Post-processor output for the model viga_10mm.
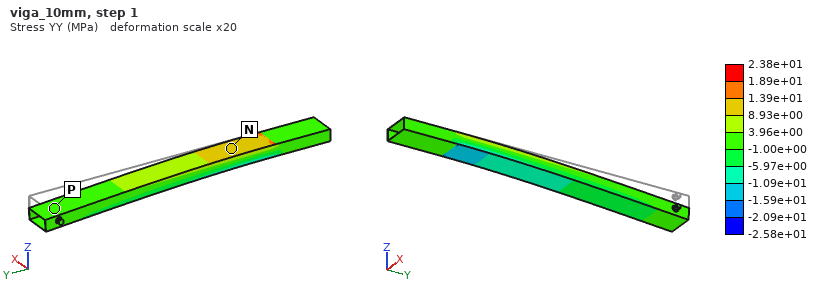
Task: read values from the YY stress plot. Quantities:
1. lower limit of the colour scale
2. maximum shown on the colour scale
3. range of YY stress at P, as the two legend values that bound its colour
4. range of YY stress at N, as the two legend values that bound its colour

-2.58e+01 MPa
2.38e+01 MPa
-1.00e+00 to 3.96e+00 MPa
8.93e+00 to 1.39e+01 MPa
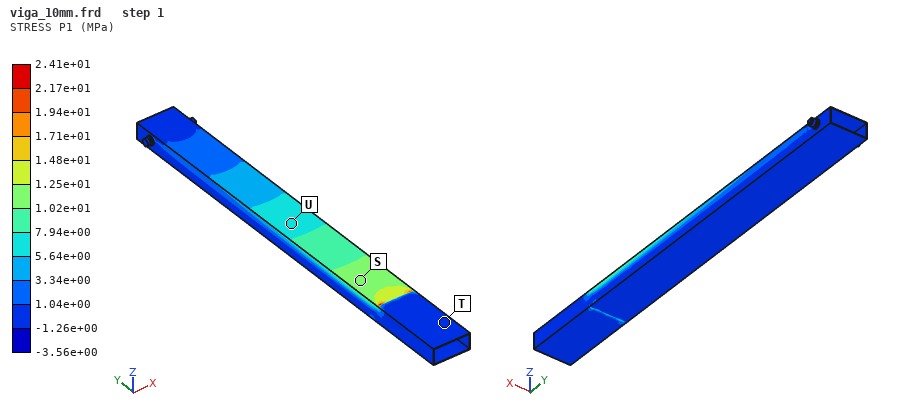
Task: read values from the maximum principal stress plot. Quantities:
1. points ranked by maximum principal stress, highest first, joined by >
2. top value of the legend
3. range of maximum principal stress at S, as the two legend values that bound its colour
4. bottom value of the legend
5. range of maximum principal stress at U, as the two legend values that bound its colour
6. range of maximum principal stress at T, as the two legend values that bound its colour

S > U > T
2.41e+01 MPa
1.02e+01 to 1.25e+01 MPa
-3.56e+00 MPa
5.64e+00 to 7.94e+00 MPa
-1.26e+00 to 1.04e+00 MPa
